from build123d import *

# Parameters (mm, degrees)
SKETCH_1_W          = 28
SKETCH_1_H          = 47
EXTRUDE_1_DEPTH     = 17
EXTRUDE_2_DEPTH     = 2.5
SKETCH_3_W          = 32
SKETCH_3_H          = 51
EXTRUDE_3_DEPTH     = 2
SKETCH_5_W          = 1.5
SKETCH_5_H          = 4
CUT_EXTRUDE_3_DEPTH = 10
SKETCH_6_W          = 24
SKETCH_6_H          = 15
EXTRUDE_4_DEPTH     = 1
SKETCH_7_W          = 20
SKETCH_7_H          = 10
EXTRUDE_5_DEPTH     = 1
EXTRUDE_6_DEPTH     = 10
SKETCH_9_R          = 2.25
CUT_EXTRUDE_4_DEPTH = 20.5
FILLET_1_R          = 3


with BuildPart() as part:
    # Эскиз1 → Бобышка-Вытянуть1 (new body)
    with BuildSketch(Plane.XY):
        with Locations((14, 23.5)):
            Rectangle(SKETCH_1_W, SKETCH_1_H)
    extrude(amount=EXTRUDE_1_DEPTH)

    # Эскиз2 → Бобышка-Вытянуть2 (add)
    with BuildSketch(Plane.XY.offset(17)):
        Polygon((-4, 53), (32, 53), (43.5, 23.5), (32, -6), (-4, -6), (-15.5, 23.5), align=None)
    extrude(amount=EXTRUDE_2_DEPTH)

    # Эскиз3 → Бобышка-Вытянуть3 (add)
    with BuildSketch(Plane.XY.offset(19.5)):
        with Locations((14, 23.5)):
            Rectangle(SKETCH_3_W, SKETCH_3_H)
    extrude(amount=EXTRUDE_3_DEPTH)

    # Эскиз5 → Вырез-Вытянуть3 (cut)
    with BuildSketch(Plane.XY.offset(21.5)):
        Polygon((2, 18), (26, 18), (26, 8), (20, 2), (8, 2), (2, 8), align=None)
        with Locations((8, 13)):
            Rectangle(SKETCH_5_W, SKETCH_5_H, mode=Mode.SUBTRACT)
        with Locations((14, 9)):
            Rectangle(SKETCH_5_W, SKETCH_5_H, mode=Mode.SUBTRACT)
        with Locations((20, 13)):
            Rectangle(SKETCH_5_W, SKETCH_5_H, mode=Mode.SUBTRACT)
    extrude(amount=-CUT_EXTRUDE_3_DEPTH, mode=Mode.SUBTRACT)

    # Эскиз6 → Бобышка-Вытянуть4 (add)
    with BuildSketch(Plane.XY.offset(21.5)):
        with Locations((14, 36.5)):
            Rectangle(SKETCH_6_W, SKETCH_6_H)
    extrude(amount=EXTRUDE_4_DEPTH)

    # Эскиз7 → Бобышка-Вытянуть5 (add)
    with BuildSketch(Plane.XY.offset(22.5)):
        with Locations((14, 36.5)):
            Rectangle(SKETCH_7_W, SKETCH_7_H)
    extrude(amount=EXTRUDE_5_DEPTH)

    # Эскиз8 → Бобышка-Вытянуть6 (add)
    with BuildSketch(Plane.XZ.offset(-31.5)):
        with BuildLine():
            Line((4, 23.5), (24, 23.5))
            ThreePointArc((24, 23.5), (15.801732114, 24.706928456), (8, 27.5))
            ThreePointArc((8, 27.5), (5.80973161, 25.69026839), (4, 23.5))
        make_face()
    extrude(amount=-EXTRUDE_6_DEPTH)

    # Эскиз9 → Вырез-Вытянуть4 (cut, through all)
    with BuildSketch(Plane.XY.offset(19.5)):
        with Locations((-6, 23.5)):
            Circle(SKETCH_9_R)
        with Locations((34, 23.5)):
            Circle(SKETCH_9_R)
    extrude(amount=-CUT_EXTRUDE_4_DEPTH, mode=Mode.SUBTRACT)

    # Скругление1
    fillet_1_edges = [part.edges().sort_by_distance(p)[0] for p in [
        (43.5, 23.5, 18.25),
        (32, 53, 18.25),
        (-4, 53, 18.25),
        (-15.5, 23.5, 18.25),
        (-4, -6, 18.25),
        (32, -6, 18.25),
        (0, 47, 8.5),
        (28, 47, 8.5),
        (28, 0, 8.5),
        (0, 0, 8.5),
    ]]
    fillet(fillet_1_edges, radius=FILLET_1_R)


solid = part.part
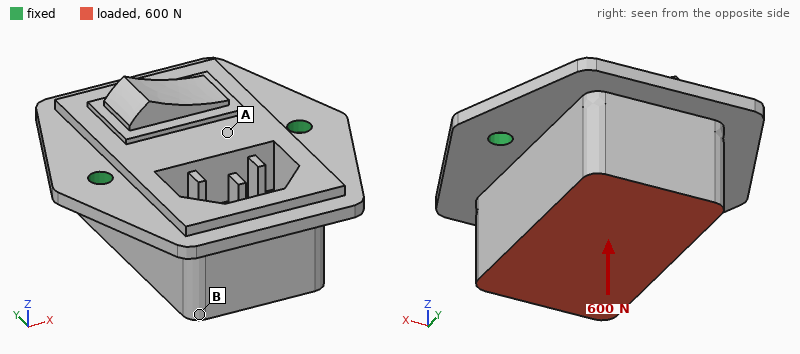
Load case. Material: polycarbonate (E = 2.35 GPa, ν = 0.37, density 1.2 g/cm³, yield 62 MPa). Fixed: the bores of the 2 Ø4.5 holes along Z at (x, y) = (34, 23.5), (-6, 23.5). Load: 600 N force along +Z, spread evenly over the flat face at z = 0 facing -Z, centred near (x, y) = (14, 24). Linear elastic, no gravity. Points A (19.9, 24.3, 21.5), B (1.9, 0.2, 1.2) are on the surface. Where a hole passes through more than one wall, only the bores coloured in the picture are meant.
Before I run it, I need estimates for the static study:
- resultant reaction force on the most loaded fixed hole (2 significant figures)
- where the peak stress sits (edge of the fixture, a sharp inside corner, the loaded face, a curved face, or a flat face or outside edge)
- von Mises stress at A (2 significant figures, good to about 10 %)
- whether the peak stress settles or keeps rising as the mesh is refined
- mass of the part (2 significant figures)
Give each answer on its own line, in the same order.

300 N
edge of the fixture
4.3 MPa
keeps rising
36 g
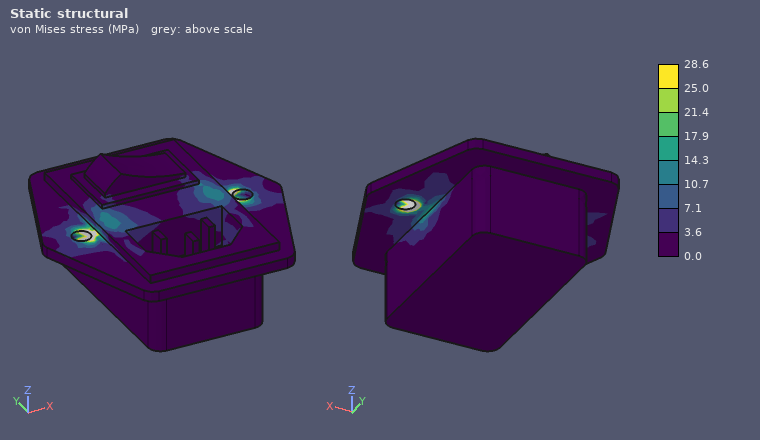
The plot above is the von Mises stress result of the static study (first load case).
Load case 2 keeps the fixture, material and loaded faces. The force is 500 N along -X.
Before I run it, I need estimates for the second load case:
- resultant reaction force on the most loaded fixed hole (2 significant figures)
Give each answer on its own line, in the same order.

360 N
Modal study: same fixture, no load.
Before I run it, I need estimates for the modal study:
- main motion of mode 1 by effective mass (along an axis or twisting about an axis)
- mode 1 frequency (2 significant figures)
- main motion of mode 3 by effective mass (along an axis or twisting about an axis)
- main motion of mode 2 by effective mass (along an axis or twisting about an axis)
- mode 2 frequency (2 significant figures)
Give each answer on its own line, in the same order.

along Y
420 Hz
along X
along Z
1700 Hz
